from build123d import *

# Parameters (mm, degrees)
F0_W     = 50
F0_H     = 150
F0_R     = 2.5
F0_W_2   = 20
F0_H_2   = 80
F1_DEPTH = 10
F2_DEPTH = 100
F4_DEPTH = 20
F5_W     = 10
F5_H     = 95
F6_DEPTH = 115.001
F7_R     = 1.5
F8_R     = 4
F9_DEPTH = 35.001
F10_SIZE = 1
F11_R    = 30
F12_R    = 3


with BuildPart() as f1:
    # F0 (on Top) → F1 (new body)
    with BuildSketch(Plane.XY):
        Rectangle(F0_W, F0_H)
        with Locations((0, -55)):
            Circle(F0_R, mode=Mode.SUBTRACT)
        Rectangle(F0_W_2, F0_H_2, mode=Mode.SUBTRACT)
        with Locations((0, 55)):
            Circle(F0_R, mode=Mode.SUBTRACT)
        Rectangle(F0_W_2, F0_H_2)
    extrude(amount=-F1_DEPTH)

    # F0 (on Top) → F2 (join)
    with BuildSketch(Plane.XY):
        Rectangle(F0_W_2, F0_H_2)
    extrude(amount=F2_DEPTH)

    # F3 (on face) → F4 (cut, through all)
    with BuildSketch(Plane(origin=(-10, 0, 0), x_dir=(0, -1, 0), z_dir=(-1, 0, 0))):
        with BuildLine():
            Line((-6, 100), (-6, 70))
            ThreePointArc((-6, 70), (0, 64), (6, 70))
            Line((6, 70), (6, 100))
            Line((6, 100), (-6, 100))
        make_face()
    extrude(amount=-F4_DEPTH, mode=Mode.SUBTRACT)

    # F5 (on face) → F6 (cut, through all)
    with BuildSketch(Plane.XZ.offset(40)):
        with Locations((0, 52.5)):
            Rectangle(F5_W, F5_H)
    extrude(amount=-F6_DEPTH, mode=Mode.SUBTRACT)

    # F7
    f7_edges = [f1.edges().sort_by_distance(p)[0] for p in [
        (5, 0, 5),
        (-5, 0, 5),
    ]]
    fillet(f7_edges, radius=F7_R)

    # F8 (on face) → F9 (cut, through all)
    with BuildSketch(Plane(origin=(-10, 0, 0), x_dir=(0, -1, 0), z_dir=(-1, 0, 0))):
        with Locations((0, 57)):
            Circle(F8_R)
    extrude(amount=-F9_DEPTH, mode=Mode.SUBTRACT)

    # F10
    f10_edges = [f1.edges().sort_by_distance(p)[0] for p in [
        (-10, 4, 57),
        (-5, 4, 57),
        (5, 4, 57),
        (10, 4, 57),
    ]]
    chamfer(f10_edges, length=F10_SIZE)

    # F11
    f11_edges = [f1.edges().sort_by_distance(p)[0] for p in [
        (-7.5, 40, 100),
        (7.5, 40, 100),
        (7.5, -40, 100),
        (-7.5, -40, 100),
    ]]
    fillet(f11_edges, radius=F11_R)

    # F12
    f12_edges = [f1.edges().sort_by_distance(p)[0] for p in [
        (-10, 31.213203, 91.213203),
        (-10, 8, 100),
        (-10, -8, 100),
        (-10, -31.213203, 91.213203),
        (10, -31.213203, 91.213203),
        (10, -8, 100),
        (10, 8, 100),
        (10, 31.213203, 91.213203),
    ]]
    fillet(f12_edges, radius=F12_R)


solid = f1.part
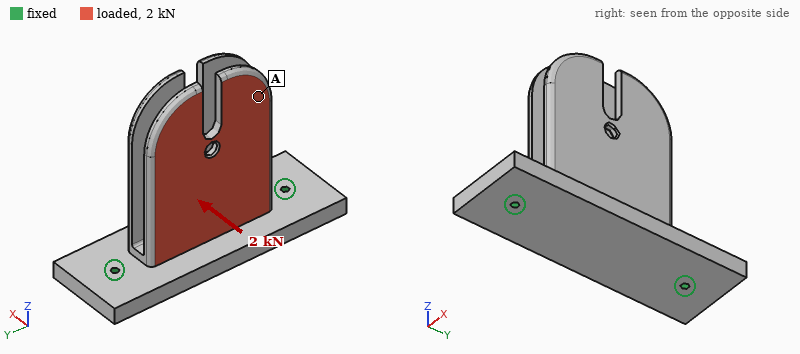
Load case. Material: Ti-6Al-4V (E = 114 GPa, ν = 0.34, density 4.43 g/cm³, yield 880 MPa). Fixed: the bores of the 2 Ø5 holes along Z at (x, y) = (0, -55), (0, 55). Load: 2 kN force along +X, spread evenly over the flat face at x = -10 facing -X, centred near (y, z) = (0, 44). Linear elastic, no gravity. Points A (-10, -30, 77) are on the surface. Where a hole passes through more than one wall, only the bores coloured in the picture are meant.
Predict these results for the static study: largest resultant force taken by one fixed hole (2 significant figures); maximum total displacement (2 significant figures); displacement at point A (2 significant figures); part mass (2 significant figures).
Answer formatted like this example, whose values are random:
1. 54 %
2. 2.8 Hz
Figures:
1. 1.0 kN
2. 2.1 mm
3. 1.4 mm
4. 660 g
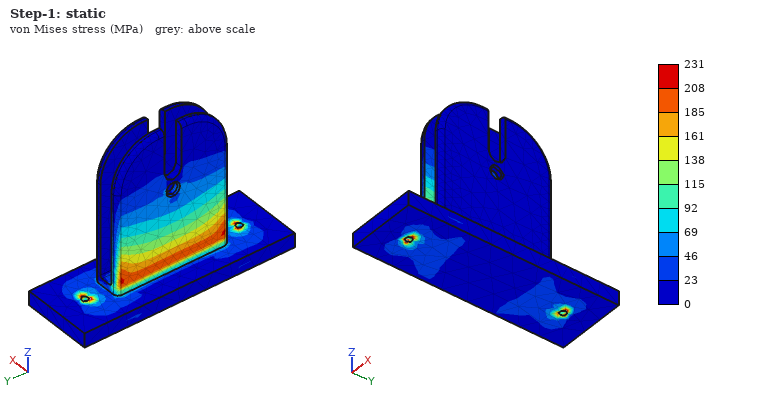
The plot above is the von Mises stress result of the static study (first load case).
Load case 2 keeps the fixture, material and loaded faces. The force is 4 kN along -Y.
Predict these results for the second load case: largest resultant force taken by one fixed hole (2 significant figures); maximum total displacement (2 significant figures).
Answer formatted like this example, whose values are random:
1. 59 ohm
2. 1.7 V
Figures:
1. 2.9 kN
2. 87 µm
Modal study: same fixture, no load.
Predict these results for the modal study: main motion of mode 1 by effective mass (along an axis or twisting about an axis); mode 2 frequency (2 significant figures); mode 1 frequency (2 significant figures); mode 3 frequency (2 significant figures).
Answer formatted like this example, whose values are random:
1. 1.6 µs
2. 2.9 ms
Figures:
1. along X
2. 530 Hz
3. 480 Hz
4. 1100 Hz
